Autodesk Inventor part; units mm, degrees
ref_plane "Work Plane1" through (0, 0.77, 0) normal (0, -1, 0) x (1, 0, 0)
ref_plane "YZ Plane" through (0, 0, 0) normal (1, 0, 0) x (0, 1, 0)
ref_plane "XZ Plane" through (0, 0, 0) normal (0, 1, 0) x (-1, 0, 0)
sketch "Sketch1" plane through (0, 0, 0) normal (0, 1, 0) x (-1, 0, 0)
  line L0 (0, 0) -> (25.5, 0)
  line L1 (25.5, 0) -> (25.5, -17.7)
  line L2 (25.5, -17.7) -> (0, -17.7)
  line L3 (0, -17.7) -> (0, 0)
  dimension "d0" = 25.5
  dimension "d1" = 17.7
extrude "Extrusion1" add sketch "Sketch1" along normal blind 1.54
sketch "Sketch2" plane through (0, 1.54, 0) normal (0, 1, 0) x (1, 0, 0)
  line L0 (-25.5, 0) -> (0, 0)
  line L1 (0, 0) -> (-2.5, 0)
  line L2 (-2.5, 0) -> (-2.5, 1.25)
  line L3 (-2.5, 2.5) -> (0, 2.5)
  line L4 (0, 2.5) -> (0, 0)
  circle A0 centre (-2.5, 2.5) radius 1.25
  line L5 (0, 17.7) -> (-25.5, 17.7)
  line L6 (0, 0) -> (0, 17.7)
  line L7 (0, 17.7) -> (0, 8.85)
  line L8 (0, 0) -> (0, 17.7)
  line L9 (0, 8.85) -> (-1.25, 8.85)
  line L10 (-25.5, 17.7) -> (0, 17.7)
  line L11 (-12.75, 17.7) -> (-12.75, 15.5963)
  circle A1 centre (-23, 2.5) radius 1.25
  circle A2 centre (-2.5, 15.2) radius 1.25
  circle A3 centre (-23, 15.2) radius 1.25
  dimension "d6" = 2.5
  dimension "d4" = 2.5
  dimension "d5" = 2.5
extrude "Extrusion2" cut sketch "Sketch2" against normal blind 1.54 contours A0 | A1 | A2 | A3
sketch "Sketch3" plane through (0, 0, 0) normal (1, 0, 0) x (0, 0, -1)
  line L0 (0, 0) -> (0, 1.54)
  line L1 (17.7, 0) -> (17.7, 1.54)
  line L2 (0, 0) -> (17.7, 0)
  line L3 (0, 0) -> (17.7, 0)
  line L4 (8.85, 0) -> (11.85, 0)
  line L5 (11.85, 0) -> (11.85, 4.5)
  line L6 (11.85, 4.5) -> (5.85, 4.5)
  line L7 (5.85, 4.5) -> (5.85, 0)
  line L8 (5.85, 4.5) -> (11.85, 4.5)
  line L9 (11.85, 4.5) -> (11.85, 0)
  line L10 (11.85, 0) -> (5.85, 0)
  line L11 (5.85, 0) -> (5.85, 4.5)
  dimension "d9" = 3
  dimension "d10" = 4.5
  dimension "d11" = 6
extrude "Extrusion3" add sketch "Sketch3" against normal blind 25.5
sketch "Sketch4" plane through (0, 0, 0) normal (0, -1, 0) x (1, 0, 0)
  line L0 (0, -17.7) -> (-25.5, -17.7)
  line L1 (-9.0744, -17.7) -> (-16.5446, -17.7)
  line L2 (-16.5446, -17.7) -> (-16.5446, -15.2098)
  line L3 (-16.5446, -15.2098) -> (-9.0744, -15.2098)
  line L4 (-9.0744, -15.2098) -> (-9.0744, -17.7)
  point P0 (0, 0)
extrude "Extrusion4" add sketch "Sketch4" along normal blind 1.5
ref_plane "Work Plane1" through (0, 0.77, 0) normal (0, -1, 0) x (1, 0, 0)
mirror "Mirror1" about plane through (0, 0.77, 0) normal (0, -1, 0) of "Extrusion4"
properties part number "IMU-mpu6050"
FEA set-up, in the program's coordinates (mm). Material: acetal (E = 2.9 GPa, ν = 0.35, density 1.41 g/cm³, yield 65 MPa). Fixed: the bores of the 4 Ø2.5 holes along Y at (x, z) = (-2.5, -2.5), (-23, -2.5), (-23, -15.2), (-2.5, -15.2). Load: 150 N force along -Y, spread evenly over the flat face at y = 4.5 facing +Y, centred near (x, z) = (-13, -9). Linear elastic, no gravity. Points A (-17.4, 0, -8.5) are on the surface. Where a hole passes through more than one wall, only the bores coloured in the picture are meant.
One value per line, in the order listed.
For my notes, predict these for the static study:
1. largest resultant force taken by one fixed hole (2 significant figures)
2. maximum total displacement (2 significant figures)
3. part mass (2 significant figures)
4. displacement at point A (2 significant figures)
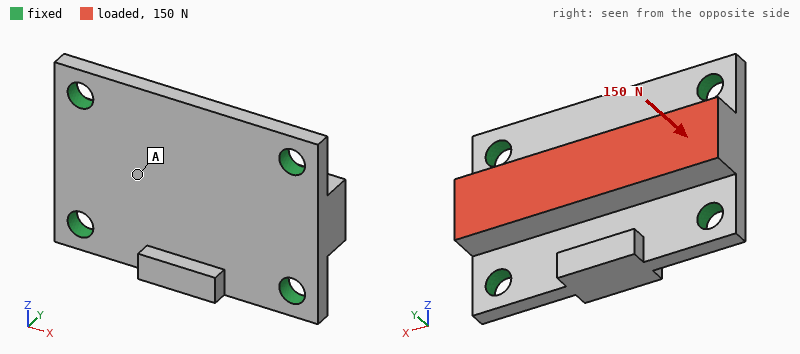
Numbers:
43 N
69 µm
1.7 g
57 µm
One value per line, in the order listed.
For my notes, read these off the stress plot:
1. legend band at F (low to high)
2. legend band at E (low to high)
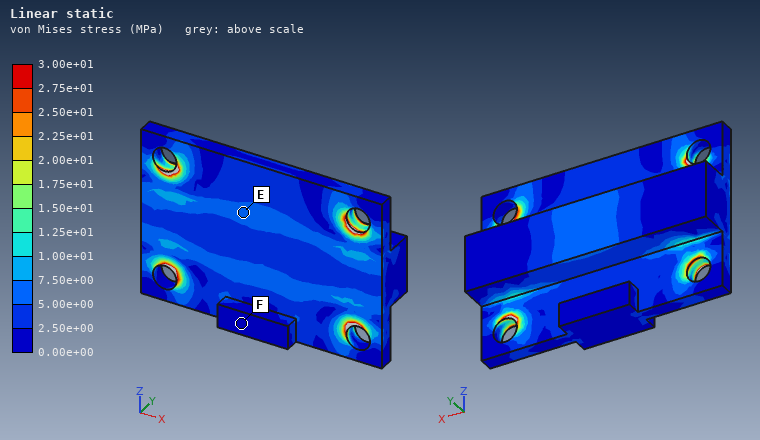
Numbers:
0.00e+00 to 2.50e+00 MPa
5.00e+00 to 7.50e+00 MPa
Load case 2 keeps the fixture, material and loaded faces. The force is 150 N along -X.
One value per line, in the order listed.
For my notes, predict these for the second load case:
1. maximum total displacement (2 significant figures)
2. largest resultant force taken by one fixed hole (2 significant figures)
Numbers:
32 µm
43 N
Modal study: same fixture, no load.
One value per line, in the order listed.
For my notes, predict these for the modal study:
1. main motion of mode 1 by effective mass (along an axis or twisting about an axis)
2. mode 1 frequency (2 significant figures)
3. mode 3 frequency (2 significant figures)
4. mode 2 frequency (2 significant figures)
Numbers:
along Y
6700 Hz
11 kHz
8100 Hz
